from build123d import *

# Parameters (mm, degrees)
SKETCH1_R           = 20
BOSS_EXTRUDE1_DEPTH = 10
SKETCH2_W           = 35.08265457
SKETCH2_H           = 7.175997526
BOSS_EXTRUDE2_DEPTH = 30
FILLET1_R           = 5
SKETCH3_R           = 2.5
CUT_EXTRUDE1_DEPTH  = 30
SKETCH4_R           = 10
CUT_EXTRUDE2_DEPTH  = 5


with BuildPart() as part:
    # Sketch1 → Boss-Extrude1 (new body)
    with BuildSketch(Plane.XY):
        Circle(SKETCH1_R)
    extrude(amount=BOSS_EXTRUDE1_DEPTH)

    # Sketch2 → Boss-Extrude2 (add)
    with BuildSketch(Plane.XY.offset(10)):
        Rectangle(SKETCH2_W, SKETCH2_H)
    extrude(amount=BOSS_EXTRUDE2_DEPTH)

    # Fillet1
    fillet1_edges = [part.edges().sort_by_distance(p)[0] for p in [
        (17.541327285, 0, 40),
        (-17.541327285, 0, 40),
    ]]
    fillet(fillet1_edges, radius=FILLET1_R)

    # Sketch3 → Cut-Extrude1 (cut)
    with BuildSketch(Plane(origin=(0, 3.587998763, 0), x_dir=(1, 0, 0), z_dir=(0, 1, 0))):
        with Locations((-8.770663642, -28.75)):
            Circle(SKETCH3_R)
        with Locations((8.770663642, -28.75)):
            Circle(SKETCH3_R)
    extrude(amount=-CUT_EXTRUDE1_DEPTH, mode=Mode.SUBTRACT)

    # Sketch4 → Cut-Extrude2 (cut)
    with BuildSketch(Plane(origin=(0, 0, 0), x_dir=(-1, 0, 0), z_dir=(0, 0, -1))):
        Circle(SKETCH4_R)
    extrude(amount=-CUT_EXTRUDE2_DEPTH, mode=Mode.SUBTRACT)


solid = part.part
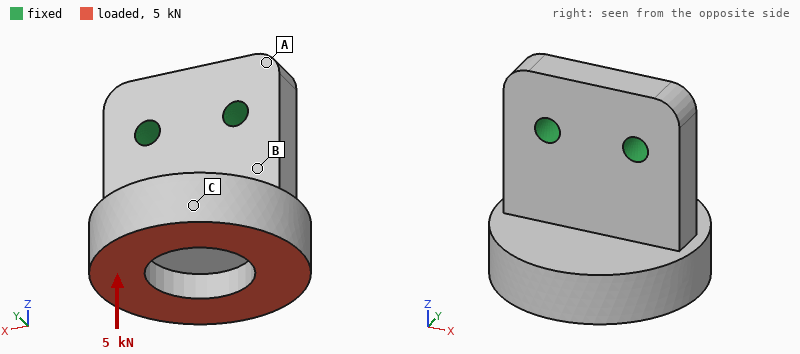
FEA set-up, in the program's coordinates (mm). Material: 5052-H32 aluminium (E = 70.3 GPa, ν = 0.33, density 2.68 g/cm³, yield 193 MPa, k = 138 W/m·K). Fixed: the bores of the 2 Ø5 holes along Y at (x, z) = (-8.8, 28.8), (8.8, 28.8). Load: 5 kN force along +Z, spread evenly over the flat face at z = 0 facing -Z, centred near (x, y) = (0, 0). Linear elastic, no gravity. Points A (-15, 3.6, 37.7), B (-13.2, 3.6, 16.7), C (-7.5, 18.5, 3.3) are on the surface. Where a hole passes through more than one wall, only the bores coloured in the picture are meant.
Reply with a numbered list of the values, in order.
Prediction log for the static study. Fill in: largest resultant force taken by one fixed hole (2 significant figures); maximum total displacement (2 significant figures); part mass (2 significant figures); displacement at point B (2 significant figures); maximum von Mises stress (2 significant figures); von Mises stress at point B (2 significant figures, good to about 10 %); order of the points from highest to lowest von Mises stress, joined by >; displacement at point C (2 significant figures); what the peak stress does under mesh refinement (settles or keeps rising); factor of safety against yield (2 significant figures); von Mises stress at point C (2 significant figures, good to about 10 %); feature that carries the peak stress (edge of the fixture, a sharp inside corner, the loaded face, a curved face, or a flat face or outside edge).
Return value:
1. 2.5 kN
2. 27 µm
3. 49 g
4. 4.2 µm
5. 65 MPa
6. 20 MPa
7. B > C > A
8. 23 µm
9. settles
10. 3.0
11. 11 MPa
12. the loaded face
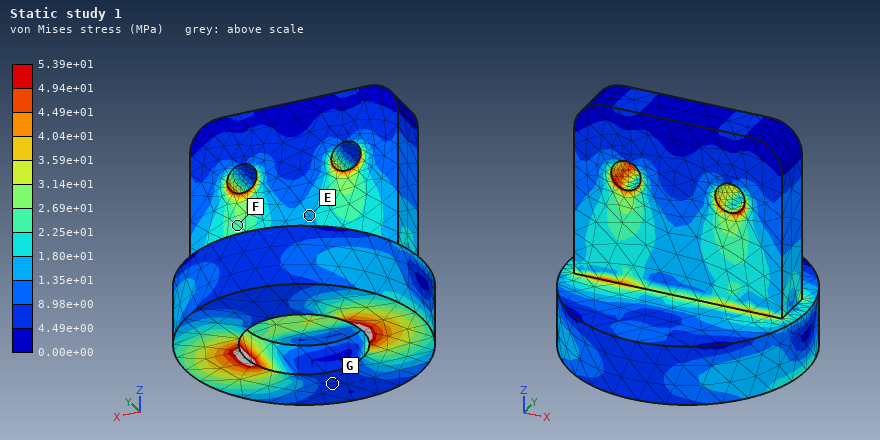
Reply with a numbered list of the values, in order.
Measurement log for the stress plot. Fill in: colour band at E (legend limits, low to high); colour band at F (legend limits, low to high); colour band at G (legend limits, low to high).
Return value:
1. 1.35e+01 to 1.80e+01 MPa
2. 2.25e+01 to 2.69e+01 MPa
3. 4.49e+00 to 8.98e+00 MPa
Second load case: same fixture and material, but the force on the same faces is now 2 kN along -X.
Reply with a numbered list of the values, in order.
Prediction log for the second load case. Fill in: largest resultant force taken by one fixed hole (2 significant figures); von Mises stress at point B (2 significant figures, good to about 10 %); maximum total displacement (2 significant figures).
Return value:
1. 2.9 kN
2. 17 MPa
3. 26 µm
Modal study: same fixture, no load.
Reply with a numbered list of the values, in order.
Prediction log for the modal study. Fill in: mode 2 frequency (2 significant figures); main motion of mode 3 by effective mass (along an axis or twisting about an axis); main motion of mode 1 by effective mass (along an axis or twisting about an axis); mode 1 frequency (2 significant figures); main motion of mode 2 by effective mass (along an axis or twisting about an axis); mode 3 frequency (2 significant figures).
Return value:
1. 6200 Hz
2. along X
3. along Y
4. 3200 Hz
5. twisting about Z
6. 9700 Hz
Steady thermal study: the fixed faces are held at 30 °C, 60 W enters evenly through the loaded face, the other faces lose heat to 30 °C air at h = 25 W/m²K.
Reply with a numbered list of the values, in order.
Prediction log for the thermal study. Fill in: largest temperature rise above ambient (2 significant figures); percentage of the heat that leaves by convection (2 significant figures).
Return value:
1. 42 K
2. 5.6 %
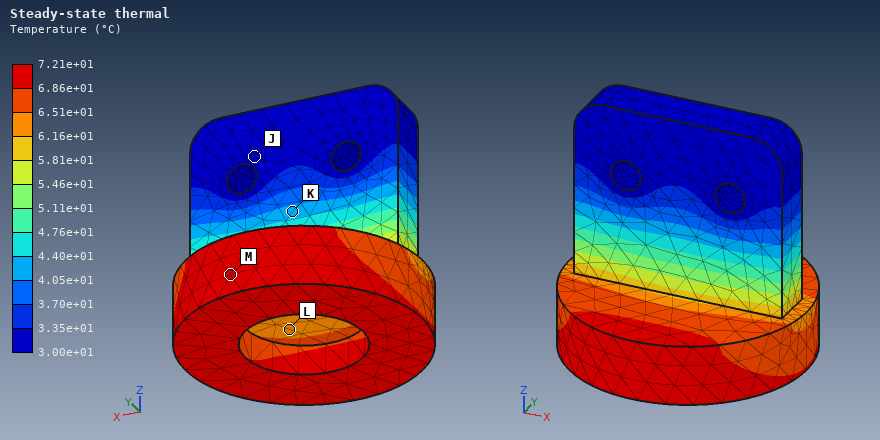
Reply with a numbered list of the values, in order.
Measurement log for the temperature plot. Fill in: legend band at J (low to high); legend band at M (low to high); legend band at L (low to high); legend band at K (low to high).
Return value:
1. 3.00e+01 to 3.35e+01 °C
2. 6.86e+01 to 7.21e+01 °C
3. 6.16e+01 to 6.51e+01 °C
4. 4.05e+01 to 4.40e+01 °C
